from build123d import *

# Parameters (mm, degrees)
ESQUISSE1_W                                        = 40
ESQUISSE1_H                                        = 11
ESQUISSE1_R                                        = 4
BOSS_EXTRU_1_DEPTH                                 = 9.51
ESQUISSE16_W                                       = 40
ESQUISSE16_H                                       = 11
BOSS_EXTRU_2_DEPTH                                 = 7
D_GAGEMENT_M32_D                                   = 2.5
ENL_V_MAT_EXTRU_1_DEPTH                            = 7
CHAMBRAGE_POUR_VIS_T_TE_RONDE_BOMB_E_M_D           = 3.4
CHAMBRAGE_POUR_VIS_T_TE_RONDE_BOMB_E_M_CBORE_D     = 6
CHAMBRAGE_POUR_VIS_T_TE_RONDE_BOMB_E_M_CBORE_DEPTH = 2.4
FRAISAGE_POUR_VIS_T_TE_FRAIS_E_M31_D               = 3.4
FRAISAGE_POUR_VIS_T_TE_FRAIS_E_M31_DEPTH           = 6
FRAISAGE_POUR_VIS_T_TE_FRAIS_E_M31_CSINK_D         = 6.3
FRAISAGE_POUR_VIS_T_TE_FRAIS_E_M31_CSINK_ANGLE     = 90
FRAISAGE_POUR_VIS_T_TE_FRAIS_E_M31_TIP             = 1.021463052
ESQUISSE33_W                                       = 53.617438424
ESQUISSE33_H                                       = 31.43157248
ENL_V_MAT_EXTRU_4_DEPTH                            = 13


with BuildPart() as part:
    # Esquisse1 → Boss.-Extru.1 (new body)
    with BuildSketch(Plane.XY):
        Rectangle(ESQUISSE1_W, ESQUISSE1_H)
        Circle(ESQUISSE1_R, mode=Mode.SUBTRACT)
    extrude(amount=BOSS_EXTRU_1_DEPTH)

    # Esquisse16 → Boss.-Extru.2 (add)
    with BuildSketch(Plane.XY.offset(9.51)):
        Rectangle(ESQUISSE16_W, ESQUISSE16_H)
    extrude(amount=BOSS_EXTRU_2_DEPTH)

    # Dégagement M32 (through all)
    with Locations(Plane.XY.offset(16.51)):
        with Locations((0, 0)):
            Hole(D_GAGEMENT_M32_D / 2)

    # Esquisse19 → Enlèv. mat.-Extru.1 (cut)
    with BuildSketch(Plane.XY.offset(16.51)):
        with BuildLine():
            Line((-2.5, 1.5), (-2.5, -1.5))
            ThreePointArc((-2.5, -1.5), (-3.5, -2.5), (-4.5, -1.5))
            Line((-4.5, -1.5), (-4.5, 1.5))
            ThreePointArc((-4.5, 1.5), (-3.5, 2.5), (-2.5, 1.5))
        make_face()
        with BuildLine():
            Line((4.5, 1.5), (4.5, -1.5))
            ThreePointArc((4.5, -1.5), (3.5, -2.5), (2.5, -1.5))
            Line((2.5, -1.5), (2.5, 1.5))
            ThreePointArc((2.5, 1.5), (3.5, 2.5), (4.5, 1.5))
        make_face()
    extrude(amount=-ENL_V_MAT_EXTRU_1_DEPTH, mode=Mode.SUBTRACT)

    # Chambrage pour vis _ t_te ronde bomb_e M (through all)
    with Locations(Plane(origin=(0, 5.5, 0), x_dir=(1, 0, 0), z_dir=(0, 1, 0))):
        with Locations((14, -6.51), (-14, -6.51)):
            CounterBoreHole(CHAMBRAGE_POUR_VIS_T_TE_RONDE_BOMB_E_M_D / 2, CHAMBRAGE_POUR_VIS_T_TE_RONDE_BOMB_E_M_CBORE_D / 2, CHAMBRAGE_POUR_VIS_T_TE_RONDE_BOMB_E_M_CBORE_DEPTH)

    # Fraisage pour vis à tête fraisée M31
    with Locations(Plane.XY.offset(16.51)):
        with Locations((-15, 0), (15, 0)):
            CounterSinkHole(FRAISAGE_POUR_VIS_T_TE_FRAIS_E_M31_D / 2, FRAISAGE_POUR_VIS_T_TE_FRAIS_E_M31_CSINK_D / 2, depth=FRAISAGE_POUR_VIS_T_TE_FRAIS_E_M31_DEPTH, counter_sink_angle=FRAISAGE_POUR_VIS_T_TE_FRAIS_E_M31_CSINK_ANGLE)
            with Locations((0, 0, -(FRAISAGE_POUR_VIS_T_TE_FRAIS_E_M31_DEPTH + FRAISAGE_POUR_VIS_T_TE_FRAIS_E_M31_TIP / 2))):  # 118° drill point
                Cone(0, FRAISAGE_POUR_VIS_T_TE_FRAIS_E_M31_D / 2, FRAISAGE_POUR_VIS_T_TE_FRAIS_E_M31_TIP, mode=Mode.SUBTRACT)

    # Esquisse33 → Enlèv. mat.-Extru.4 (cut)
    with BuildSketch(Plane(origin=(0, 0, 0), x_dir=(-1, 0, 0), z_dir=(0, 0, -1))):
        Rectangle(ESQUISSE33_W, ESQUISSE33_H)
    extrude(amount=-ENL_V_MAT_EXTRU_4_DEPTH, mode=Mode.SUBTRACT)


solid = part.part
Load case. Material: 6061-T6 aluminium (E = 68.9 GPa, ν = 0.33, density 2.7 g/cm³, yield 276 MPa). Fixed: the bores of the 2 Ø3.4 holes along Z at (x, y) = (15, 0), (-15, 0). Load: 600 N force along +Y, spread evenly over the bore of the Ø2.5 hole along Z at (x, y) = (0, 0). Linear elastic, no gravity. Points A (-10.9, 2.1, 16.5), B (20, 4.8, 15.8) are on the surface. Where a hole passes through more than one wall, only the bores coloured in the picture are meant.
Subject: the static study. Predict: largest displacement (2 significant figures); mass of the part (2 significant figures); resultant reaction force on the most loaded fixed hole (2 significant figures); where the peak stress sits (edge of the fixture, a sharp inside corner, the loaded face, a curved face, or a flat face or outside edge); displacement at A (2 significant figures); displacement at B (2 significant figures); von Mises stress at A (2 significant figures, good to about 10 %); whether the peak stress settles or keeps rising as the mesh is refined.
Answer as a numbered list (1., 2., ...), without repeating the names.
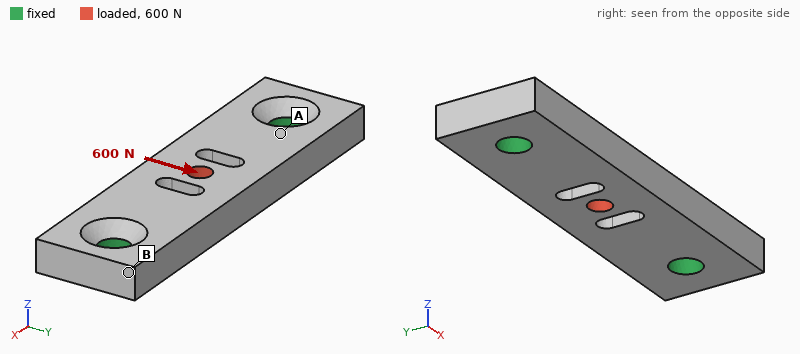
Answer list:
1. 15 µm
2. 3.7 g
3. 300 N
4. edge of the fixture
5. 4.0 µm
6. 3.0 µm
7. 17 MPa
8. keeps rising
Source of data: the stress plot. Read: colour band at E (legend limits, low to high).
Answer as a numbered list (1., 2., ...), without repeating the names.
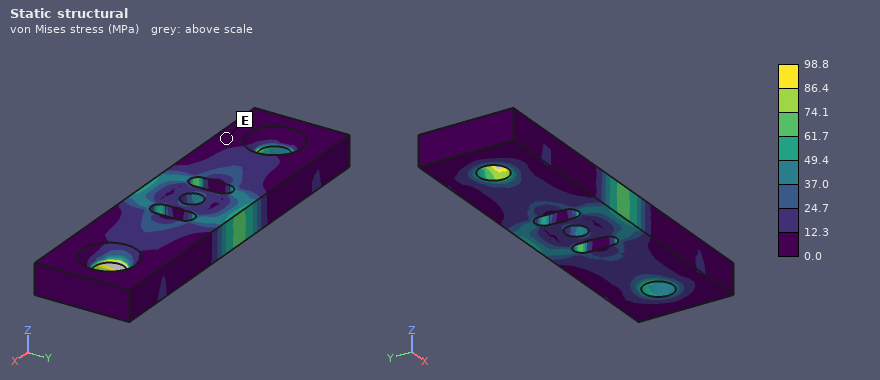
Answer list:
1. 0.0 to 12.3 MPa
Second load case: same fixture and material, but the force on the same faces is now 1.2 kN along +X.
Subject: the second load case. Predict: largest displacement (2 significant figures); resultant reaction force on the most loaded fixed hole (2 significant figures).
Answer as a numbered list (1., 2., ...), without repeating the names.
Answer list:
1. 11 µm
2. 600 N
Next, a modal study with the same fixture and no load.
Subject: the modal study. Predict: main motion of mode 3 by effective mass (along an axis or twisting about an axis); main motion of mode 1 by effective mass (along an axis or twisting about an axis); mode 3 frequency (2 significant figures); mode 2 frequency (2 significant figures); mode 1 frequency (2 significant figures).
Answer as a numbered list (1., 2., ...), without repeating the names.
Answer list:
1. along Y
2. along Z
3. 32 kHz
4. 26 kHz
5. 17 kHz
